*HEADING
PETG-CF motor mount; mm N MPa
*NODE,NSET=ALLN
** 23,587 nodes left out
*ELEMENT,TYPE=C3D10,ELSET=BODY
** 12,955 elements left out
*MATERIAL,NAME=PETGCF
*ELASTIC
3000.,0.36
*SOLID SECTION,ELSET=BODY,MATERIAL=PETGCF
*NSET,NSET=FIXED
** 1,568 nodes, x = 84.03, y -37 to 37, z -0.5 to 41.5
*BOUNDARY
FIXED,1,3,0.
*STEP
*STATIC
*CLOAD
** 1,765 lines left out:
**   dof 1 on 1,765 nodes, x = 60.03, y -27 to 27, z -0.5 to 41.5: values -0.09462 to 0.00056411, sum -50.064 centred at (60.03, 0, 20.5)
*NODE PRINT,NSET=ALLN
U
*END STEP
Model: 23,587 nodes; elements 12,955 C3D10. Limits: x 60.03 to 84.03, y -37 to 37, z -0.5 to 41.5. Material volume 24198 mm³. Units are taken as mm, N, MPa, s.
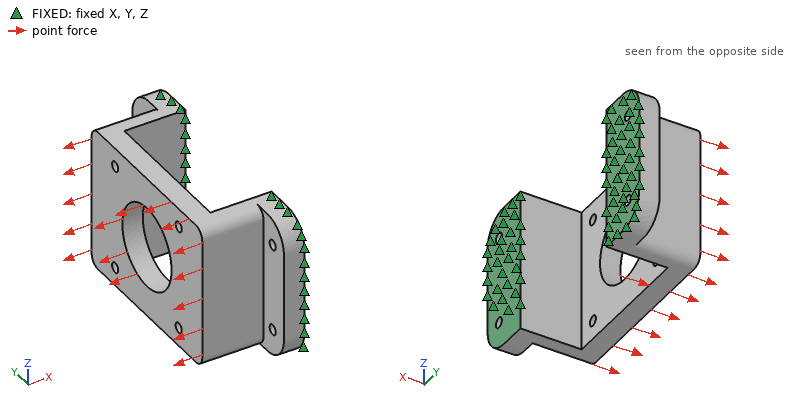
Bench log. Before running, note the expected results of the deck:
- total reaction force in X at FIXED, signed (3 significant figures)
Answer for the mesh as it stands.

50.1 N
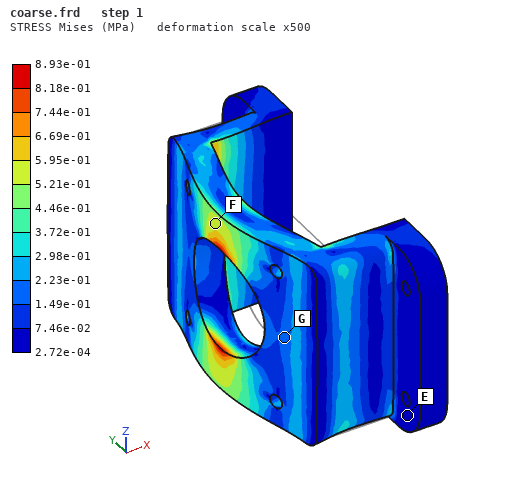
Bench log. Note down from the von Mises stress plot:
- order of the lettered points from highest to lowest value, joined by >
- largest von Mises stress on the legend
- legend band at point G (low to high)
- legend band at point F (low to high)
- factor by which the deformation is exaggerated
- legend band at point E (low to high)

F > G > E
8.93e-01 MPa
1.49e-01 to 2.23e-01 MPa
5.21e-01 to 5.95e-01 MPa
500
2.72e-04 to 7.46e-02 MPa
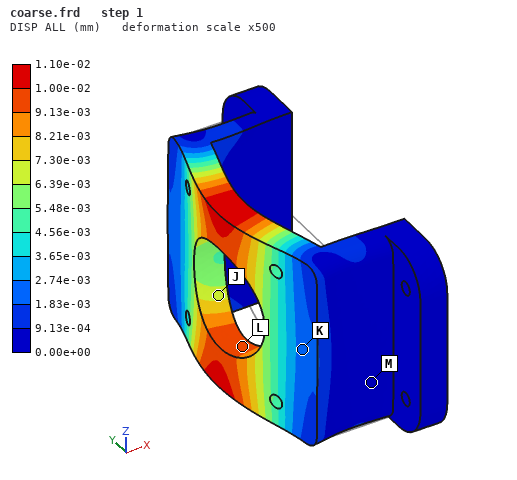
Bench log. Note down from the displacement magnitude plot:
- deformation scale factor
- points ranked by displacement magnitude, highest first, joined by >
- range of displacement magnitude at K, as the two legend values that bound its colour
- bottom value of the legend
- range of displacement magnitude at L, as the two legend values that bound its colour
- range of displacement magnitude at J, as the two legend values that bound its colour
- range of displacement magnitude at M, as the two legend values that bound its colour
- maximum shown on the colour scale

500
L > J > K > M
1.83e-03 to 2.74e-03 mm
0.00e+00 mm
9.13e-03 to 1.00e-02 mm
6.39e-03 to 7.30e-03 mm
0.00e+00 to 9.13e-04 mm
1.10e-02 mm
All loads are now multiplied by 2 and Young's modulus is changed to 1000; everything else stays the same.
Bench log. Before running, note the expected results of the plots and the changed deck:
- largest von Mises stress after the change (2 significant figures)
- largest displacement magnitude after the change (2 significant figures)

1.8 MPa
0.066 mm
